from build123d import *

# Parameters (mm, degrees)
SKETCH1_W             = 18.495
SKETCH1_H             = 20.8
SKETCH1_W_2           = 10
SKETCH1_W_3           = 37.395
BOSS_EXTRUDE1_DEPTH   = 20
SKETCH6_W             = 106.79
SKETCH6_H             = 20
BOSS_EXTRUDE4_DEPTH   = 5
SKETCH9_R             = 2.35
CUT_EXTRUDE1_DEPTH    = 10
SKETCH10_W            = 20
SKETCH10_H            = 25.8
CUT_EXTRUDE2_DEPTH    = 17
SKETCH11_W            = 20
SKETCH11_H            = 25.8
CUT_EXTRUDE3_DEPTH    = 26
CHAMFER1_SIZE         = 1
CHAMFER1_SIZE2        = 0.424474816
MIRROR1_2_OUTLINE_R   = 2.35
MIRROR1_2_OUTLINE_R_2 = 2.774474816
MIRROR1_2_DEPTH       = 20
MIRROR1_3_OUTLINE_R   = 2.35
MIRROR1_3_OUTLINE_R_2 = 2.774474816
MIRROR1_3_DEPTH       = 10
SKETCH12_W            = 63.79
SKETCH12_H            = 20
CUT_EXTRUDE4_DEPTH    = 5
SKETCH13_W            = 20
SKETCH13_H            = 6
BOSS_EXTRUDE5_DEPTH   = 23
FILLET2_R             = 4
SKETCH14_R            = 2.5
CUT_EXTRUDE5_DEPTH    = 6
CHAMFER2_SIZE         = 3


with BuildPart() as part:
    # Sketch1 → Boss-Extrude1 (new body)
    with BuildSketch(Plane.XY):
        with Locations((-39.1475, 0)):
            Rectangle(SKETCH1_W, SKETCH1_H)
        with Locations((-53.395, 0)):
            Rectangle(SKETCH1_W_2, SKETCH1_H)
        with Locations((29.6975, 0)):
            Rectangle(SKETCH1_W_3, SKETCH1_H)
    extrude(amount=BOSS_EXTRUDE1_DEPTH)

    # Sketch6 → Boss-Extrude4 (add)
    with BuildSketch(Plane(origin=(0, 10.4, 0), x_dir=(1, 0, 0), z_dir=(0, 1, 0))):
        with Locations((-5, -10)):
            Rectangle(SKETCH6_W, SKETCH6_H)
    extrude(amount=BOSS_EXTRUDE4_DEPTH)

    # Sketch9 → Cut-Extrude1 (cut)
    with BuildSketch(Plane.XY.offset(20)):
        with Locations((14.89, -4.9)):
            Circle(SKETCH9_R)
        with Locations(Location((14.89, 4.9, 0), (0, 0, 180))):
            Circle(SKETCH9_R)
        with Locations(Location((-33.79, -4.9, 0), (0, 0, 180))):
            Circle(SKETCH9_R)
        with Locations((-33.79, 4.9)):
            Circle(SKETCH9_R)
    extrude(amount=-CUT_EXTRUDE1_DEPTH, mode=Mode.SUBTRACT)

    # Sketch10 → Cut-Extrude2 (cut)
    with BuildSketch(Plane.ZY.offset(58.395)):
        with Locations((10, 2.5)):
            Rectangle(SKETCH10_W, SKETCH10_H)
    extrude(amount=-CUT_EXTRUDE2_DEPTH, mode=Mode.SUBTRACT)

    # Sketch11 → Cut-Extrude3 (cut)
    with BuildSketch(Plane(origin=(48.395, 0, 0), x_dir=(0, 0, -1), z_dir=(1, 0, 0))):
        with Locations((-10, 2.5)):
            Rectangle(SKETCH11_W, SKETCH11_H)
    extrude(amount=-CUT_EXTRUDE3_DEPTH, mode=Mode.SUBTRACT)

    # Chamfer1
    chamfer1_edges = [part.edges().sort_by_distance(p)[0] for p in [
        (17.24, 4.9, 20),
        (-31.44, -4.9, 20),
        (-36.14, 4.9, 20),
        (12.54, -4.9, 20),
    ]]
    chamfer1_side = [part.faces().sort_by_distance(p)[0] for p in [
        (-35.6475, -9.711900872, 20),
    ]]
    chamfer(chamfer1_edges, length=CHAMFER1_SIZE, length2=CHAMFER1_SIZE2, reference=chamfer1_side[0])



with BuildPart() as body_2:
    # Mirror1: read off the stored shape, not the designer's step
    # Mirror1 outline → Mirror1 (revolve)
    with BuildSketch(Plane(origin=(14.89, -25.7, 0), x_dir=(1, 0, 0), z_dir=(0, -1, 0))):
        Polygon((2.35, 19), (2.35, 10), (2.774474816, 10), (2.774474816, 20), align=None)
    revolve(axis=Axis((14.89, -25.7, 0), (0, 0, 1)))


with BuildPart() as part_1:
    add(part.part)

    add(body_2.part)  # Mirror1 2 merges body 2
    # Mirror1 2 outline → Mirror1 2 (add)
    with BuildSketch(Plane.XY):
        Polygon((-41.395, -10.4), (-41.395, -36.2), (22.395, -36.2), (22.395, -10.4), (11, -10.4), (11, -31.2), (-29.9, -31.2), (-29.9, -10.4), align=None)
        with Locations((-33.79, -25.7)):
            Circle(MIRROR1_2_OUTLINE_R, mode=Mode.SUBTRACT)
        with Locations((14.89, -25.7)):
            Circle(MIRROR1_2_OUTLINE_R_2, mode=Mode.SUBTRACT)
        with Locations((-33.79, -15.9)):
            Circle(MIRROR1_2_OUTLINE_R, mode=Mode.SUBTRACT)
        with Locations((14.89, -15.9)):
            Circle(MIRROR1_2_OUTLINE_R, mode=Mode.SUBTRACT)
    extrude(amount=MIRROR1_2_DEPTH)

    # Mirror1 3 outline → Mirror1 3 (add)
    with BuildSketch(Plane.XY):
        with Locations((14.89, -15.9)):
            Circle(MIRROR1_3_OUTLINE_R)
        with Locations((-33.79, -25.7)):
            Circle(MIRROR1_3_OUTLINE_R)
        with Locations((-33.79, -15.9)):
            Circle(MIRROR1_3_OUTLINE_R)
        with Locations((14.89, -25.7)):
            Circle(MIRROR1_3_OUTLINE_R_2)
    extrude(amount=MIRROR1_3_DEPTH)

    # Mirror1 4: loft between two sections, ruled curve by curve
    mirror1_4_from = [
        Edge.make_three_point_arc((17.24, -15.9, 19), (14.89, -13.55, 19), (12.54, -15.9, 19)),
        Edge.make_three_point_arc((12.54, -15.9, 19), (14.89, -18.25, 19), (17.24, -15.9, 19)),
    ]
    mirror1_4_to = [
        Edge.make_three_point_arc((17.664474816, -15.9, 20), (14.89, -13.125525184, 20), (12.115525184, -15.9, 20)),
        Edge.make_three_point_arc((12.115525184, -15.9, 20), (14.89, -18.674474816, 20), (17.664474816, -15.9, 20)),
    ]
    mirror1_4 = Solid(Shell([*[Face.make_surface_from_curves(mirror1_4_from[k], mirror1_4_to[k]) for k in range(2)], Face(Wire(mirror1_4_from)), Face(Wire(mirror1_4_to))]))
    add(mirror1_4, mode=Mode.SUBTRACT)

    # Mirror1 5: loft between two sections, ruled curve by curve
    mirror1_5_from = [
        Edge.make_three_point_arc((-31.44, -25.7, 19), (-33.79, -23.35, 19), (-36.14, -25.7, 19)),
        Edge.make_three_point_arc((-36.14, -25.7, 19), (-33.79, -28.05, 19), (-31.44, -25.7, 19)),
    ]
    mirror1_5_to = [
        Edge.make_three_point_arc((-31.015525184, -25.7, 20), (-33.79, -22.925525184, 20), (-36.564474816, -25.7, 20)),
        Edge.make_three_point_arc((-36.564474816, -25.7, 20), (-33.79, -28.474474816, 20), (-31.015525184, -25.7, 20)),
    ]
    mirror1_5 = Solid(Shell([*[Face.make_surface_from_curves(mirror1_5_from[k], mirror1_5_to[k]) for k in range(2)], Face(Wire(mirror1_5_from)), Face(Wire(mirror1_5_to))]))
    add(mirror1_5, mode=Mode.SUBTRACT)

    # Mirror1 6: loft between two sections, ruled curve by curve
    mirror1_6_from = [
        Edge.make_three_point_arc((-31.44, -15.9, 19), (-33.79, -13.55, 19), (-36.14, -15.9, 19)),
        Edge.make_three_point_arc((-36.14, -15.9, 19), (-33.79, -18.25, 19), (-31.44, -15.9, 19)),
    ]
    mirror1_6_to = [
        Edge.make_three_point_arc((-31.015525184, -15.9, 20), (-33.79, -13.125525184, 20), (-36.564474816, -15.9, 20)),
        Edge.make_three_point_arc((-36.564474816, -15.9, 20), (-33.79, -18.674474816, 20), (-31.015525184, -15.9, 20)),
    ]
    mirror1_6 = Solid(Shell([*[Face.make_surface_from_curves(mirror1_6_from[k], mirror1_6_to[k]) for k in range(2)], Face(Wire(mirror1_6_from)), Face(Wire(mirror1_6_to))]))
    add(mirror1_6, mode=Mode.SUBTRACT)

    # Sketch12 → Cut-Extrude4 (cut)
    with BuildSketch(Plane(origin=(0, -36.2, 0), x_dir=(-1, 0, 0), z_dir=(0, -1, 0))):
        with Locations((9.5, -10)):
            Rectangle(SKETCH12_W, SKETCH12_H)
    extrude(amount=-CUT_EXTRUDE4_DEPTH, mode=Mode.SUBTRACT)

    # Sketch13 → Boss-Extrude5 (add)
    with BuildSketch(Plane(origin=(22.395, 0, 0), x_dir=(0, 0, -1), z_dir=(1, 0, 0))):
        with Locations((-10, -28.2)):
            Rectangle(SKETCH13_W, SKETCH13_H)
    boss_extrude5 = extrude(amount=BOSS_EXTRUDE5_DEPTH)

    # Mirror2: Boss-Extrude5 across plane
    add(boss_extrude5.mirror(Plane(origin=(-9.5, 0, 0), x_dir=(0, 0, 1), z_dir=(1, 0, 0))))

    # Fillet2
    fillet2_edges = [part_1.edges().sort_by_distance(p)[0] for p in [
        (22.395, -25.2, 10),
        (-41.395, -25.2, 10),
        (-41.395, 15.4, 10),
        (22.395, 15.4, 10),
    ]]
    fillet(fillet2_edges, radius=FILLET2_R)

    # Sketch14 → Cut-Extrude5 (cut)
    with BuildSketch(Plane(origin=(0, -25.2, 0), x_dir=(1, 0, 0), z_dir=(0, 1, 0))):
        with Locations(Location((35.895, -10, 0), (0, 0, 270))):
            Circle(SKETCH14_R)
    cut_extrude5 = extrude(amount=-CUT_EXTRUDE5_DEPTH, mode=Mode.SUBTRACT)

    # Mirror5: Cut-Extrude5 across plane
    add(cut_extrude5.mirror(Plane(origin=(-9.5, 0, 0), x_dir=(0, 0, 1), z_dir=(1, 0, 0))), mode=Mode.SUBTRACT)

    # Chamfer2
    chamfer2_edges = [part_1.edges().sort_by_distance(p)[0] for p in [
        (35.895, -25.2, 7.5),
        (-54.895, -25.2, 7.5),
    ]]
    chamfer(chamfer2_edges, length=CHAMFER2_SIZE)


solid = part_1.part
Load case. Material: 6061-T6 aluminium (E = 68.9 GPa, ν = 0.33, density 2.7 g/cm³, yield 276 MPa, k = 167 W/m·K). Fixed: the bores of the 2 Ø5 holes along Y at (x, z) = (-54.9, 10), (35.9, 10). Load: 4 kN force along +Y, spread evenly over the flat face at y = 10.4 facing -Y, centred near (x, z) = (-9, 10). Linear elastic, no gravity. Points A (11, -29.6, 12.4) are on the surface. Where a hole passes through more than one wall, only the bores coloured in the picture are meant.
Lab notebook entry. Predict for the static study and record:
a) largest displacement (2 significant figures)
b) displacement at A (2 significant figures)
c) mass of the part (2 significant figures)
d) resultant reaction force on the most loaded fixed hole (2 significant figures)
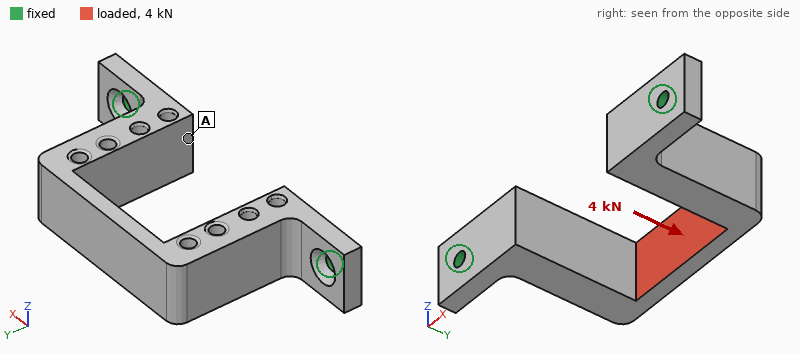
0.16 mm
0.058 mm
79 g
2.3 kN
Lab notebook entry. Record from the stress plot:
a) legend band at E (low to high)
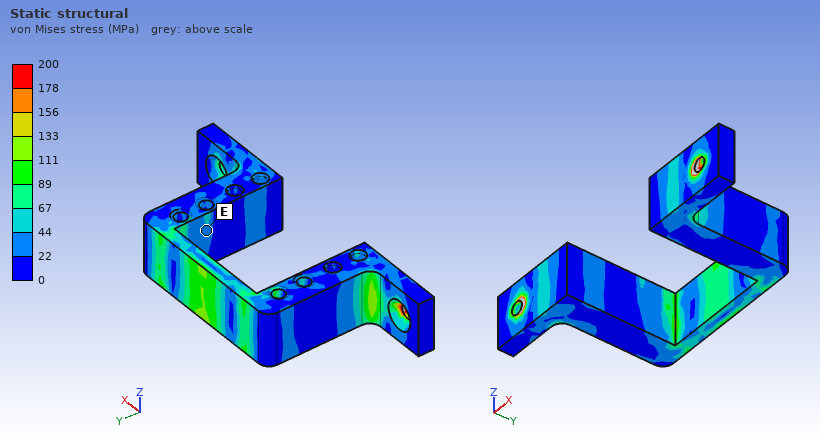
22 to 44 MPa
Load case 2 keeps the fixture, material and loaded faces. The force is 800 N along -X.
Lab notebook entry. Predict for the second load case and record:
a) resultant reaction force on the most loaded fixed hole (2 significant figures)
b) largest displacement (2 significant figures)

500 N
0.13 mm
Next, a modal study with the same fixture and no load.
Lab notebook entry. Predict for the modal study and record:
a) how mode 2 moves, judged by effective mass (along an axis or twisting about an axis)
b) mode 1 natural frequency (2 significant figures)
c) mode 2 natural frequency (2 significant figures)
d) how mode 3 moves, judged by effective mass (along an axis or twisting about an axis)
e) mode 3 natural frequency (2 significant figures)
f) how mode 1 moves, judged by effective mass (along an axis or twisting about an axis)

along X
1200 Hz
2200 Hz
twisting about Y
3300 Hz
along Z
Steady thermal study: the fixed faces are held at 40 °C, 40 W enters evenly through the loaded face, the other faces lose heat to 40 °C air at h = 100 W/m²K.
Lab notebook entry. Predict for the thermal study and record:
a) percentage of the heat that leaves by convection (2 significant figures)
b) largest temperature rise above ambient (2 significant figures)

45 %
40 K
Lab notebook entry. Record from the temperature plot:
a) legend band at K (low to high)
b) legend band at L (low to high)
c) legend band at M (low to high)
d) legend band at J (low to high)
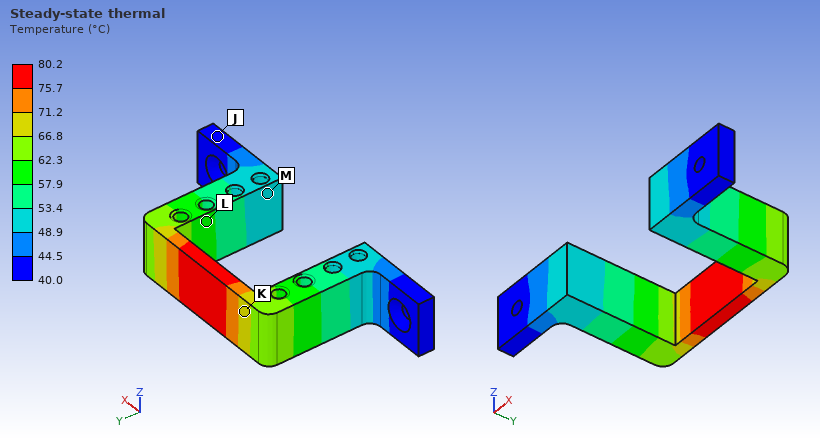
66.8 to 71.2 °C
57.9 to 62.3 °C
48.9 to 53.4 °C
40.0 to 44.5 °C
